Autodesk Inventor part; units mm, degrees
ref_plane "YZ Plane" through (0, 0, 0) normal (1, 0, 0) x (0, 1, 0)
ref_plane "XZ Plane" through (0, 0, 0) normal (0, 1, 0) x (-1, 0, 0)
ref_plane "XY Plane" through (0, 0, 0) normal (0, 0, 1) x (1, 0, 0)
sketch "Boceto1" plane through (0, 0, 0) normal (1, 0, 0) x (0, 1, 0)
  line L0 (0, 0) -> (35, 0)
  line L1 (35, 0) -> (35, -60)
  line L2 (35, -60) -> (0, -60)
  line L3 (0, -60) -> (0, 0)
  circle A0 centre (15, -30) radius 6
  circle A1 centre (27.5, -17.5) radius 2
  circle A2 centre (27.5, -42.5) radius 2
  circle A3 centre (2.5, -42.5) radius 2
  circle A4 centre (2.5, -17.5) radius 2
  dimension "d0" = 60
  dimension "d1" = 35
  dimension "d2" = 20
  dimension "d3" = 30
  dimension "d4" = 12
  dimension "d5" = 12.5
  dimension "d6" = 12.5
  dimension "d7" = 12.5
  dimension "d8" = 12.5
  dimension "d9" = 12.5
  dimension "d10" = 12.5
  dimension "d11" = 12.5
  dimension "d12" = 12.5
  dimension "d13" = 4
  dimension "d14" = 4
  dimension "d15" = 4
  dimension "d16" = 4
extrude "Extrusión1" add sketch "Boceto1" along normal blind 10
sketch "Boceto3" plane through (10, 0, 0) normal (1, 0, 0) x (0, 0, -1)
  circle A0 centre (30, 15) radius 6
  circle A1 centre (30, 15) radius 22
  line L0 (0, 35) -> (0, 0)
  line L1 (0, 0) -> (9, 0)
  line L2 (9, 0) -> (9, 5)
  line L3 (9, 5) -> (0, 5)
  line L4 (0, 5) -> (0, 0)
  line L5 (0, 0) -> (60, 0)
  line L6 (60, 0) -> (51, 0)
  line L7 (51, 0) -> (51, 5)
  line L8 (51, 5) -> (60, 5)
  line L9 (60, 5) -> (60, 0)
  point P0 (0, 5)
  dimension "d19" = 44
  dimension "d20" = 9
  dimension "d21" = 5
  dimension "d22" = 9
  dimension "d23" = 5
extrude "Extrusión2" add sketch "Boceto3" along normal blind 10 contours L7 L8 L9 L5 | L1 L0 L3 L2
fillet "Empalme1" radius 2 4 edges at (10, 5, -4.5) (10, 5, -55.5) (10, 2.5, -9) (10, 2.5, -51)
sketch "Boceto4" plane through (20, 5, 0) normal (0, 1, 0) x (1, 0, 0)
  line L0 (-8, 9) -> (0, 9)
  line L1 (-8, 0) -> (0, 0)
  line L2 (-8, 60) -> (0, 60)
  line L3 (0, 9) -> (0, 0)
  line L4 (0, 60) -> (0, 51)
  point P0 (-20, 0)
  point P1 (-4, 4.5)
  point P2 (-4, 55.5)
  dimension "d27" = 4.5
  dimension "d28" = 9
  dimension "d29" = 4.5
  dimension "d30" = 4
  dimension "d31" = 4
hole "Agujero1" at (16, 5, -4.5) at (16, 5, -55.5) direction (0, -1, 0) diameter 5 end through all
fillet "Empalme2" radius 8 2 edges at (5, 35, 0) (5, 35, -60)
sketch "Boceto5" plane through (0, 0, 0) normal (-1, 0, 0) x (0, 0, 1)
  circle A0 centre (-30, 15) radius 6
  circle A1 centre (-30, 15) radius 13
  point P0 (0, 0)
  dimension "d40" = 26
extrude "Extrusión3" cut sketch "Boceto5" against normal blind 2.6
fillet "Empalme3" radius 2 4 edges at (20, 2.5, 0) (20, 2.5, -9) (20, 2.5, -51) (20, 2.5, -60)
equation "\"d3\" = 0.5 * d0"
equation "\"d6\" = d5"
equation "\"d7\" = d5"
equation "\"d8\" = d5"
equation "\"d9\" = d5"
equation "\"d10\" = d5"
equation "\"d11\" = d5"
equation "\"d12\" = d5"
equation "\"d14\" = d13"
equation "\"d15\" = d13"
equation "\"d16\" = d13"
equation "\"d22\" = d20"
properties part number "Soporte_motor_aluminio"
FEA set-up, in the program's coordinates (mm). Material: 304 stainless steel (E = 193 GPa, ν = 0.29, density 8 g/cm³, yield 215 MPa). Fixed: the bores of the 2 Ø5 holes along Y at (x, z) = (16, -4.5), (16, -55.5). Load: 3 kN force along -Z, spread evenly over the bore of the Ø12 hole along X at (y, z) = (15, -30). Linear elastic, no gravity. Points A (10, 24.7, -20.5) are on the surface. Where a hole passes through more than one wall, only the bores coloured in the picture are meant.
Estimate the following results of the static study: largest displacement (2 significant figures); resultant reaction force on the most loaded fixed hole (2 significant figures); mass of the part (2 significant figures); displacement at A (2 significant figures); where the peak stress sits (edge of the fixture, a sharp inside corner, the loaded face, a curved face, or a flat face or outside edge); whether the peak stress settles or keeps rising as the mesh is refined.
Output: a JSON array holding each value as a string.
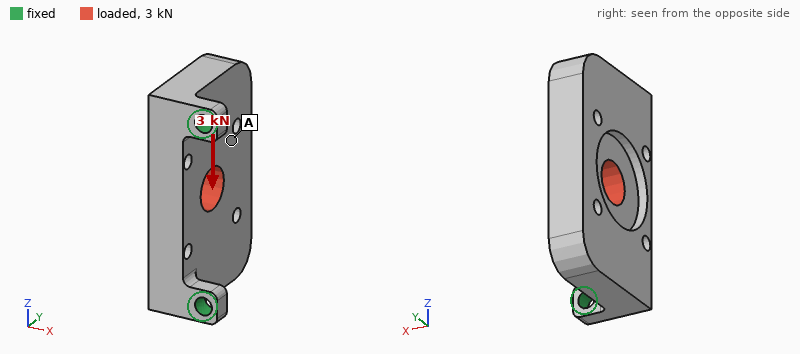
["12 µm", "1.7 kN", "150 g", "10 µm", "edge of the fixture", "keeps rising"]
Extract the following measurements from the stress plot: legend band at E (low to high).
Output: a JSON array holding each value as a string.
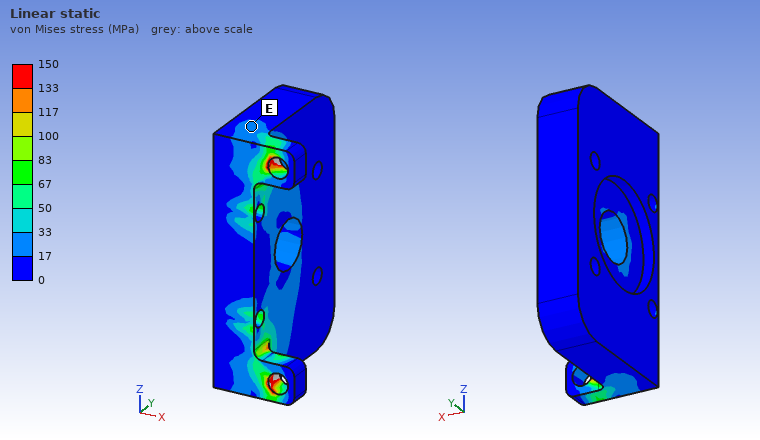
["17 to 33 MPa"]
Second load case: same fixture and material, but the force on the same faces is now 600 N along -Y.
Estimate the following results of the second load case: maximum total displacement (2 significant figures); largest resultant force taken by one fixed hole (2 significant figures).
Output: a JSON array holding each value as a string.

["17 µm", "300 N"]
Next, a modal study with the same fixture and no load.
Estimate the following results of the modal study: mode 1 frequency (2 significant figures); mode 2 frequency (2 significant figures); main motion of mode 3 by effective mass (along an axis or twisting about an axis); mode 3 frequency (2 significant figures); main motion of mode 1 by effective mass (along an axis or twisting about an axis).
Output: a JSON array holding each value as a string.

["1700 Hz", "5800 Hz", "along Z", "7900 Hz", "along X"]
